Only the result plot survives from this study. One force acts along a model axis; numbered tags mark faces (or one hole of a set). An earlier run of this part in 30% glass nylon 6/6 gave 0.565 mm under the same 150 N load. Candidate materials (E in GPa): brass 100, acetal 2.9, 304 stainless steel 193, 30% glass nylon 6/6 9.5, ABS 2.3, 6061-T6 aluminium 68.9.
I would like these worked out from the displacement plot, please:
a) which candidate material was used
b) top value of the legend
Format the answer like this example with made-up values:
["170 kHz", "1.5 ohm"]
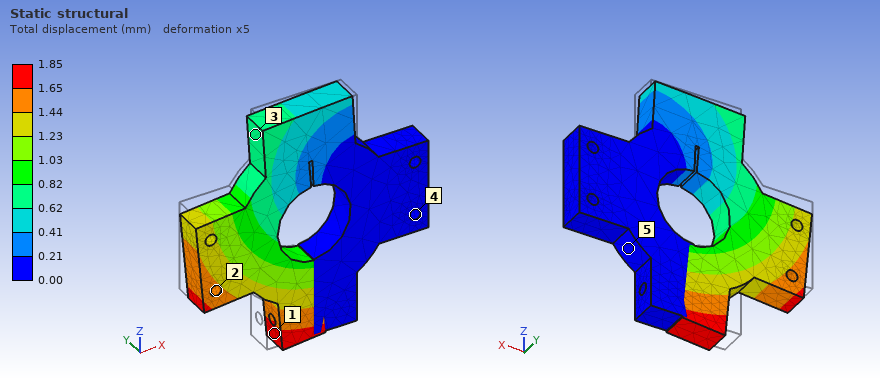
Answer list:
["acetal", "1.85 mm"]
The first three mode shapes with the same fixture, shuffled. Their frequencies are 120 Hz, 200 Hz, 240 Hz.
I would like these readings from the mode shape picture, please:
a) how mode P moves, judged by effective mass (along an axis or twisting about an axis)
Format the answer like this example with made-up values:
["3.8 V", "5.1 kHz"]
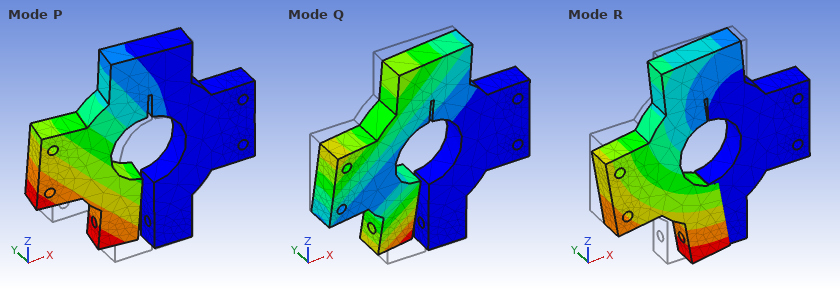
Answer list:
["along Y"]
